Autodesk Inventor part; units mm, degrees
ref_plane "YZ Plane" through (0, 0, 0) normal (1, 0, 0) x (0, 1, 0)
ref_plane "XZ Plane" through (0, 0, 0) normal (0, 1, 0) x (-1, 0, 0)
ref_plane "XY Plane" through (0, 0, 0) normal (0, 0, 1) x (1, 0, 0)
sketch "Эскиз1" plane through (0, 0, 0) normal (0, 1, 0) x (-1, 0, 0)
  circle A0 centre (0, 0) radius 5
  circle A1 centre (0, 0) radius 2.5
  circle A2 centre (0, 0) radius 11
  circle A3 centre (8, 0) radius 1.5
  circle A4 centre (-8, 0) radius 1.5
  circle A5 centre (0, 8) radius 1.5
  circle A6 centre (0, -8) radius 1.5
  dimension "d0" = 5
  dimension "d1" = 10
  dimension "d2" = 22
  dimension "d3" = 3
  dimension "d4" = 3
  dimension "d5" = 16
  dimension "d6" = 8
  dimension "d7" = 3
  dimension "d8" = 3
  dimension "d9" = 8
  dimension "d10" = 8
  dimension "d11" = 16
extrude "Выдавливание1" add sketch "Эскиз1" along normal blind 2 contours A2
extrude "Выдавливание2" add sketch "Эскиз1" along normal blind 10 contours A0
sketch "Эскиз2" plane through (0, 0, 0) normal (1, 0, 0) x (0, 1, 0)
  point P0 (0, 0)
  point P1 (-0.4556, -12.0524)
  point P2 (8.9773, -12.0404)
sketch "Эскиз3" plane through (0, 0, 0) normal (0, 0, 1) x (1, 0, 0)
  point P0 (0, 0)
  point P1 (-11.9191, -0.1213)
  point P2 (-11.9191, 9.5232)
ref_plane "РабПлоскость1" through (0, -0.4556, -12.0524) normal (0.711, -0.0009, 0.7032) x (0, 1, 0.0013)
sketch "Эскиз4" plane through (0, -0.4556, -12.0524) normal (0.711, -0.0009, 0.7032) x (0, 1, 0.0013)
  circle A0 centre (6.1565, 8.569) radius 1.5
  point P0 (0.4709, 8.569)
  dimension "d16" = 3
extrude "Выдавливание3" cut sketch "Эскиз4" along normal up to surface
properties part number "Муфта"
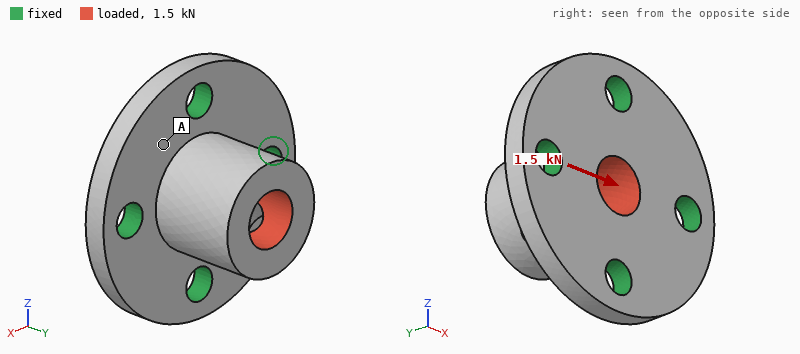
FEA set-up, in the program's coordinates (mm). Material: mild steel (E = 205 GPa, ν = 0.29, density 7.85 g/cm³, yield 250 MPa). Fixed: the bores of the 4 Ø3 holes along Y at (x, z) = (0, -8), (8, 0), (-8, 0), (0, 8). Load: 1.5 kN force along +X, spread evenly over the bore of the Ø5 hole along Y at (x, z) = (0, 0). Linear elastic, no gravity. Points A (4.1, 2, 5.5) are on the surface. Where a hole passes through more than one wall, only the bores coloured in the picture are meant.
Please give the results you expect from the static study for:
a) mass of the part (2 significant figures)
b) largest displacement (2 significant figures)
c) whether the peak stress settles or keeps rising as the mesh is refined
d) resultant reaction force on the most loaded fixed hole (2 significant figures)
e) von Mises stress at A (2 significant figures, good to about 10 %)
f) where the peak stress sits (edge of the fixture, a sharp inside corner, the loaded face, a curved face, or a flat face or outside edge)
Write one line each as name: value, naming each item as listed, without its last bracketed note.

mass of the part: 8.8 g
largest displacement: 7.6 µm
whether the peak stress settles or keeps rising as the mesh is refined: keeps rising
resultant reaction force on the most loaded fixed hole: 680 N
von Mises stress at A: 22 MPa
where the peak stress sits: edge of the fixture
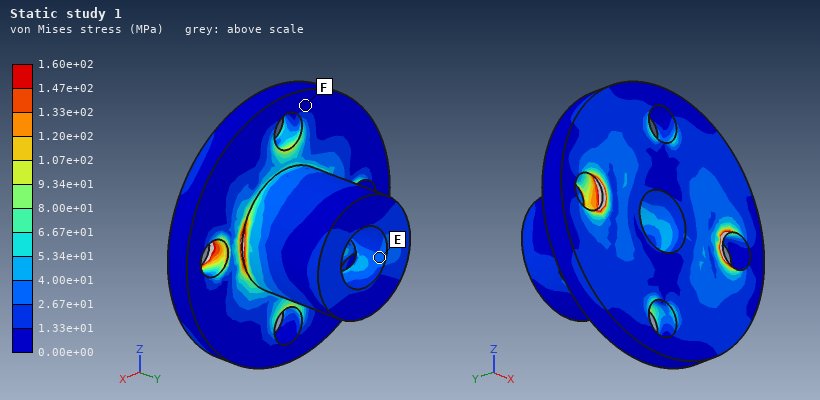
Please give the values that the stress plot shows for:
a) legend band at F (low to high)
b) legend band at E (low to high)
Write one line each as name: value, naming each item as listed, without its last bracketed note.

legend band at F: 0.00e+00 to 1.33e+01 MPa
legend band at E: 2.67e+01 to 4.00e+01 MPa
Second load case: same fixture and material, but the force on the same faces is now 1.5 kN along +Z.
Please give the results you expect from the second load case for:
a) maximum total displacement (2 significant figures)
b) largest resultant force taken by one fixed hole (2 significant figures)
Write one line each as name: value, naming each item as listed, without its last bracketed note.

maximum total displacement: 7.6 µm
largest resultant force taken by one fixed hole: 680 N
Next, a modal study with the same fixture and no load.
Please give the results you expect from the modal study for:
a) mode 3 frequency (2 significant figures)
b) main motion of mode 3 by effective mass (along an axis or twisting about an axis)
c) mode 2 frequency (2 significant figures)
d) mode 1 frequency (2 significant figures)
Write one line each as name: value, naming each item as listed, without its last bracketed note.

mode 3 frequency: 56 kHz
main motion of mode 3 by effective mass: along Y
mode 2 frequency: 39 kHz
mode 1 frequency: 38 kHz
